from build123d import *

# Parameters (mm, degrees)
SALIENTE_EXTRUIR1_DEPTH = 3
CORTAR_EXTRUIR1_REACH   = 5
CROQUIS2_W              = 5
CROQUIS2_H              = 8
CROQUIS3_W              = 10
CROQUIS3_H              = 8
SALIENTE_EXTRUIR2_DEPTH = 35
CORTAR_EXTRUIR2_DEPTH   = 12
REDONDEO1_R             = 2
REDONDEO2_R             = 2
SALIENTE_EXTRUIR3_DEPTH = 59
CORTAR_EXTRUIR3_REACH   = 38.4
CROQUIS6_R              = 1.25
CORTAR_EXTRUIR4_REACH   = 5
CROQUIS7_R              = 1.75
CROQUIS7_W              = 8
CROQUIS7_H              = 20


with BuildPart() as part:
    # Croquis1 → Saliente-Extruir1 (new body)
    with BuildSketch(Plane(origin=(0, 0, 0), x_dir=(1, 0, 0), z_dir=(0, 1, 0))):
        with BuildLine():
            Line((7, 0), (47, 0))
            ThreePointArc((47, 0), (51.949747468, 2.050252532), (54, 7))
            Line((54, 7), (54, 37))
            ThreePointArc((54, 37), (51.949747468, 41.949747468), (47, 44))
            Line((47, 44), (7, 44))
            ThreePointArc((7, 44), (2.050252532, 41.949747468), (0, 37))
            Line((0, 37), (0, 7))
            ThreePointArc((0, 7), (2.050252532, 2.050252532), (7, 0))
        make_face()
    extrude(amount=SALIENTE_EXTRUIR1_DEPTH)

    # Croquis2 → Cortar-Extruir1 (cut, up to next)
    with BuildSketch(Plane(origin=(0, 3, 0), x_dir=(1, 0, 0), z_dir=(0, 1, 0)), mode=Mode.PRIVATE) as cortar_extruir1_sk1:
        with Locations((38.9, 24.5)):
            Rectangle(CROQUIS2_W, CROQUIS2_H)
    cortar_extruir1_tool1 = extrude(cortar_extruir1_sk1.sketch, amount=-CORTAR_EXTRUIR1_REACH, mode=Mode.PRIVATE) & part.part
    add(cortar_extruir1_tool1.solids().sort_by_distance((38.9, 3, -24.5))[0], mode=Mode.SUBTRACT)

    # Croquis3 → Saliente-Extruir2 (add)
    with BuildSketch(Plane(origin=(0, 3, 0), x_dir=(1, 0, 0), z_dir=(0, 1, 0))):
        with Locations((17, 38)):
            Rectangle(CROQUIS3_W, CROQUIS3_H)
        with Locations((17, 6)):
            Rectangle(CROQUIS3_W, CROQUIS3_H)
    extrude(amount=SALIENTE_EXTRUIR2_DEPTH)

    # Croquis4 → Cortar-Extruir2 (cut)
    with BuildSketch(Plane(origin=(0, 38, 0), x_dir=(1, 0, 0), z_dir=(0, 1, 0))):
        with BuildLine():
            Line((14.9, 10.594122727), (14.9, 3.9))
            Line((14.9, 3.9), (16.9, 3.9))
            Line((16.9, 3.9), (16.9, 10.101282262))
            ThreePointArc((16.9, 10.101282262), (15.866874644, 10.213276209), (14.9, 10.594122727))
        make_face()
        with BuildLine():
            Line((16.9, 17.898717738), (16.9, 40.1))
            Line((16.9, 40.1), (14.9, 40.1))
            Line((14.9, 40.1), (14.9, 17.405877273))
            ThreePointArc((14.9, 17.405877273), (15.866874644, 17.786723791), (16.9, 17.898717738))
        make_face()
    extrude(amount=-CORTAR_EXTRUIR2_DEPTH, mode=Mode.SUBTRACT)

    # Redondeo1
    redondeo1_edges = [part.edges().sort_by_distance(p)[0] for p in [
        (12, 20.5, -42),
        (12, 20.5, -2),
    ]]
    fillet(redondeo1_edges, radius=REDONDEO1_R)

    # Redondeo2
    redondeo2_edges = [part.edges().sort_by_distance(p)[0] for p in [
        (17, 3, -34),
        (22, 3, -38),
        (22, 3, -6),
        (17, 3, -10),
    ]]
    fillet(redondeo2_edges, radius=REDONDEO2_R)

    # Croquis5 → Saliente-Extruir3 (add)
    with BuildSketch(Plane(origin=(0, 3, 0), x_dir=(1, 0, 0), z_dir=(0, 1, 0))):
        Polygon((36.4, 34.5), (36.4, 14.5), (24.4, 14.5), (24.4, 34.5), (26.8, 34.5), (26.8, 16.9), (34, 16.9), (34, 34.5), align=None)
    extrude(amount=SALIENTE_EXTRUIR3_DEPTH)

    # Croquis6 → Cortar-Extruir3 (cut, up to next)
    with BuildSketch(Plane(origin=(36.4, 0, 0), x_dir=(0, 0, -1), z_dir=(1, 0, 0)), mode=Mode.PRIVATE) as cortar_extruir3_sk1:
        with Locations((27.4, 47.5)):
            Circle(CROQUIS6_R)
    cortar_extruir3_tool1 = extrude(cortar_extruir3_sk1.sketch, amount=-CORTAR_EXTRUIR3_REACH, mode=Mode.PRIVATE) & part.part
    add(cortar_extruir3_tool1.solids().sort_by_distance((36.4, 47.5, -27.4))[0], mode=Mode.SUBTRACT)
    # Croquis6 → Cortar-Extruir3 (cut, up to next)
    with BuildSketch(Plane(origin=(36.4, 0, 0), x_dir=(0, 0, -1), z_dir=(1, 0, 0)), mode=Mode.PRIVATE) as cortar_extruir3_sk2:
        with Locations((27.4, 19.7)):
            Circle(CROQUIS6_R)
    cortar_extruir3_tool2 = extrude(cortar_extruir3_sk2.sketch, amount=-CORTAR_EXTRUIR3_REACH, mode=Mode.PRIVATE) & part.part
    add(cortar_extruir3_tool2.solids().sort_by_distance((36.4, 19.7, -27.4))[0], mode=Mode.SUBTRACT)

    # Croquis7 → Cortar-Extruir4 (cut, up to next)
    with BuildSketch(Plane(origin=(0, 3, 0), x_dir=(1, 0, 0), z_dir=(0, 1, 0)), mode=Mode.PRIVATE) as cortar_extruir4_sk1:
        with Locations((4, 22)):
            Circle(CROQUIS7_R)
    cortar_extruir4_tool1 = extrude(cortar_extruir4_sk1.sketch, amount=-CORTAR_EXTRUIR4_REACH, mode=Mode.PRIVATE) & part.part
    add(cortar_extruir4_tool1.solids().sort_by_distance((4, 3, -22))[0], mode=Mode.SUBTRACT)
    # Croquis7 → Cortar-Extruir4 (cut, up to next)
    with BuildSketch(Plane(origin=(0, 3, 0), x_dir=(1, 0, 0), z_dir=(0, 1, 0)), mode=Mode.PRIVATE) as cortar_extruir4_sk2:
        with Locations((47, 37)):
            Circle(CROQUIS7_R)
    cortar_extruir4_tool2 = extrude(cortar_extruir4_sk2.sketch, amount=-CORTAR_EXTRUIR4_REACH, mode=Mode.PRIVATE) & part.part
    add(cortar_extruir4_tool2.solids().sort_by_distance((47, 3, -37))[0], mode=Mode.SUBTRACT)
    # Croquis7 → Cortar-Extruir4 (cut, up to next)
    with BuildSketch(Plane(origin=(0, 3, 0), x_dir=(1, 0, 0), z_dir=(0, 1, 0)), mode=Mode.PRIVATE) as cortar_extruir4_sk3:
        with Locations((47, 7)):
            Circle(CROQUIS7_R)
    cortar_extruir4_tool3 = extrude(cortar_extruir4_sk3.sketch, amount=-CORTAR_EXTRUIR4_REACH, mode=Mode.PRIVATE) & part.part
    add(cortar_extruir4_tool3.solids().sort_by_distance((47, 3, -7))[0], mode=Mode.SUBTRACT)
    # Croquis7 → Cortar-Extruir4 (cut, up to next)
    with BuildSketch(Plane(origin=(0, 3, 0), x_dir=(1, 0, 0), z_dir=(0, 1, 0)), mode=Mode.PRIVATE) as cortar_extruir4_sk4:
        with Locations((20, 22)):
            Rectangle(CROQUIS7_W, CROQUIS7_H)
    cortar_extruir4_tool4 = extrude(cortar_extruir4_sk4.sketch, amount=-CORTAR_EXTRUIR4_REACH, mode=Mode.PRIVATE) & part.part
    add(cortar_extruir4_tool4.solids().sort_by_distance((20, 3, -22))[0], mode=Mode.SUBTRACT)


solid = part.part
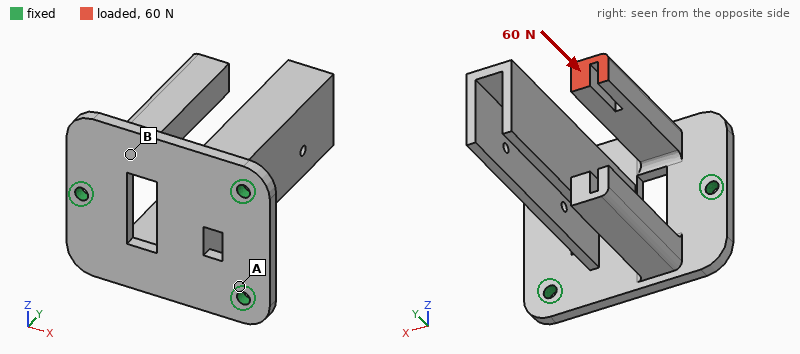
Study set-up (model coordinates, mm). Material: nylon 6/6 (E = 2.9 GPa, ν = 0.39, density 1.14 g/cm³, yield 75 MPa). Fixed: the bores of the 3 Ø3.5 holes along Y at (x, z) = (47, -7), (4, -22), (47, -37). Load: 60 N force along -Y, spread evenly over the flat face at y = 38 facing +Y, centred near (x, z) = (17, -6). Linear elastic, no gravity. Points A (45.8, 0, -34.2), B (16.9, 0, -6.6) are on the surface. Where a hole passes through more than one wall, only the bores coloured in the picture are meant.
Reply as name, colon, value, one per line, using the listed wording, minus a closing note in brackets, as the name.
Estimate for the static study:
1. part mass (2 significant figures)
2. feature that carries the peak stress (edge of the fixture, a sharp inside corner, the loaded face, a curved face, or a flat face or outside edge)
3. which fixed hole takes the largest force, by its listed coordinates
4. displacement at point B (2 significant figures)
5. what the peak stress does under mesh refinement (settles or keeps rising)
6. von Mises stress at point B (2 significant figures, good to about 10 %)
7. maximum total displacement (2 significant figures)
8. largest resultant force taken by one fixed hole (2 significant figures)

part mass: 21 g
feature that carries the peak stress: edge of the fixture
which fixed hole takes the largest force, by its listed coordinates: (4, -22)
displacement at point B: 0.32 mm
what the peak stress does under mesh refinement: keeps rising
von Mises stress at point B: 3.7 MPa
maximum total displacement: 0.99 mm
largest resultant force taken by one fixed hole: 40 N
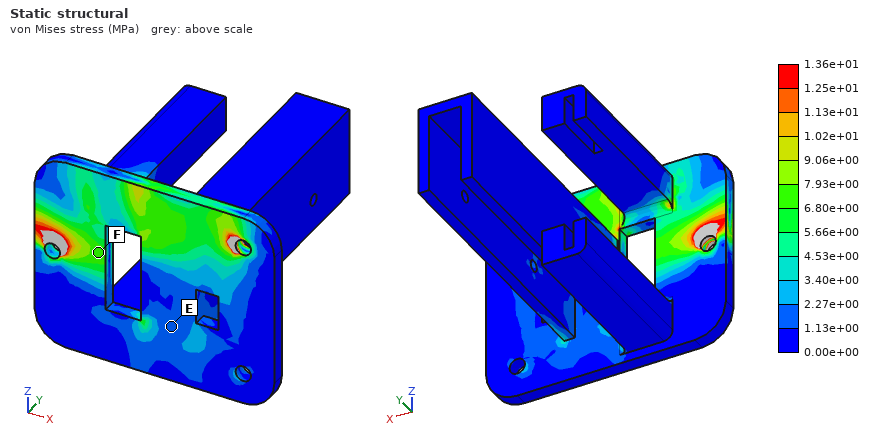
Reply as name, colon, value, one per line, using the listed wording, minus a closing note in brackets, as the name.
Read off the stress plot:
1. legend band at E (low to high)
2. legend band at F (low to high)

legend band at E: 1.13e+00 to 2.27e+00 MPa
legend band at F: 6.80e+00 to 7.93e+00 MPa
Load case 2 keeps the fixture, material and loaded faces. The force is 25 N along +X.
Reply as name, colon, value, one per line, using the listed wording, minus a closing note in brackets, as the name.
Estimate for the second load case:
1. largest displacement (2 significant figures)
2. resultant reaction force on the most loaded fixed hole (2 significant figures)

largest displacement: 1.1 mm
resultant reaction force on the most loaded fixed hole: 28 N
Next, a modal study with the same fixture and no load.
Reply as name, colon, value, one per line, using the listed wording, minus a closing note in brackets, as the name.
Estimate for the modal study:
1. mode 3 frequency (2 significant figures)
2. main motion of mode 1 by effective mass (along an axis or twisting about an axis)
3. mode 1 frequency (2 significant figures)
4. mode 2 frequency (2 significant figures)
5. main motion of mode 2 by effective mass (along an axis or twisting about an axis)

mode 3 frequency: 520 Hz
main motion of mode 1 by effective mass: along X
mode 1 frequency: 320 Hz
mode 2 frequency: 440 Hz
main motion of mode 2 by effective mass: along Z
